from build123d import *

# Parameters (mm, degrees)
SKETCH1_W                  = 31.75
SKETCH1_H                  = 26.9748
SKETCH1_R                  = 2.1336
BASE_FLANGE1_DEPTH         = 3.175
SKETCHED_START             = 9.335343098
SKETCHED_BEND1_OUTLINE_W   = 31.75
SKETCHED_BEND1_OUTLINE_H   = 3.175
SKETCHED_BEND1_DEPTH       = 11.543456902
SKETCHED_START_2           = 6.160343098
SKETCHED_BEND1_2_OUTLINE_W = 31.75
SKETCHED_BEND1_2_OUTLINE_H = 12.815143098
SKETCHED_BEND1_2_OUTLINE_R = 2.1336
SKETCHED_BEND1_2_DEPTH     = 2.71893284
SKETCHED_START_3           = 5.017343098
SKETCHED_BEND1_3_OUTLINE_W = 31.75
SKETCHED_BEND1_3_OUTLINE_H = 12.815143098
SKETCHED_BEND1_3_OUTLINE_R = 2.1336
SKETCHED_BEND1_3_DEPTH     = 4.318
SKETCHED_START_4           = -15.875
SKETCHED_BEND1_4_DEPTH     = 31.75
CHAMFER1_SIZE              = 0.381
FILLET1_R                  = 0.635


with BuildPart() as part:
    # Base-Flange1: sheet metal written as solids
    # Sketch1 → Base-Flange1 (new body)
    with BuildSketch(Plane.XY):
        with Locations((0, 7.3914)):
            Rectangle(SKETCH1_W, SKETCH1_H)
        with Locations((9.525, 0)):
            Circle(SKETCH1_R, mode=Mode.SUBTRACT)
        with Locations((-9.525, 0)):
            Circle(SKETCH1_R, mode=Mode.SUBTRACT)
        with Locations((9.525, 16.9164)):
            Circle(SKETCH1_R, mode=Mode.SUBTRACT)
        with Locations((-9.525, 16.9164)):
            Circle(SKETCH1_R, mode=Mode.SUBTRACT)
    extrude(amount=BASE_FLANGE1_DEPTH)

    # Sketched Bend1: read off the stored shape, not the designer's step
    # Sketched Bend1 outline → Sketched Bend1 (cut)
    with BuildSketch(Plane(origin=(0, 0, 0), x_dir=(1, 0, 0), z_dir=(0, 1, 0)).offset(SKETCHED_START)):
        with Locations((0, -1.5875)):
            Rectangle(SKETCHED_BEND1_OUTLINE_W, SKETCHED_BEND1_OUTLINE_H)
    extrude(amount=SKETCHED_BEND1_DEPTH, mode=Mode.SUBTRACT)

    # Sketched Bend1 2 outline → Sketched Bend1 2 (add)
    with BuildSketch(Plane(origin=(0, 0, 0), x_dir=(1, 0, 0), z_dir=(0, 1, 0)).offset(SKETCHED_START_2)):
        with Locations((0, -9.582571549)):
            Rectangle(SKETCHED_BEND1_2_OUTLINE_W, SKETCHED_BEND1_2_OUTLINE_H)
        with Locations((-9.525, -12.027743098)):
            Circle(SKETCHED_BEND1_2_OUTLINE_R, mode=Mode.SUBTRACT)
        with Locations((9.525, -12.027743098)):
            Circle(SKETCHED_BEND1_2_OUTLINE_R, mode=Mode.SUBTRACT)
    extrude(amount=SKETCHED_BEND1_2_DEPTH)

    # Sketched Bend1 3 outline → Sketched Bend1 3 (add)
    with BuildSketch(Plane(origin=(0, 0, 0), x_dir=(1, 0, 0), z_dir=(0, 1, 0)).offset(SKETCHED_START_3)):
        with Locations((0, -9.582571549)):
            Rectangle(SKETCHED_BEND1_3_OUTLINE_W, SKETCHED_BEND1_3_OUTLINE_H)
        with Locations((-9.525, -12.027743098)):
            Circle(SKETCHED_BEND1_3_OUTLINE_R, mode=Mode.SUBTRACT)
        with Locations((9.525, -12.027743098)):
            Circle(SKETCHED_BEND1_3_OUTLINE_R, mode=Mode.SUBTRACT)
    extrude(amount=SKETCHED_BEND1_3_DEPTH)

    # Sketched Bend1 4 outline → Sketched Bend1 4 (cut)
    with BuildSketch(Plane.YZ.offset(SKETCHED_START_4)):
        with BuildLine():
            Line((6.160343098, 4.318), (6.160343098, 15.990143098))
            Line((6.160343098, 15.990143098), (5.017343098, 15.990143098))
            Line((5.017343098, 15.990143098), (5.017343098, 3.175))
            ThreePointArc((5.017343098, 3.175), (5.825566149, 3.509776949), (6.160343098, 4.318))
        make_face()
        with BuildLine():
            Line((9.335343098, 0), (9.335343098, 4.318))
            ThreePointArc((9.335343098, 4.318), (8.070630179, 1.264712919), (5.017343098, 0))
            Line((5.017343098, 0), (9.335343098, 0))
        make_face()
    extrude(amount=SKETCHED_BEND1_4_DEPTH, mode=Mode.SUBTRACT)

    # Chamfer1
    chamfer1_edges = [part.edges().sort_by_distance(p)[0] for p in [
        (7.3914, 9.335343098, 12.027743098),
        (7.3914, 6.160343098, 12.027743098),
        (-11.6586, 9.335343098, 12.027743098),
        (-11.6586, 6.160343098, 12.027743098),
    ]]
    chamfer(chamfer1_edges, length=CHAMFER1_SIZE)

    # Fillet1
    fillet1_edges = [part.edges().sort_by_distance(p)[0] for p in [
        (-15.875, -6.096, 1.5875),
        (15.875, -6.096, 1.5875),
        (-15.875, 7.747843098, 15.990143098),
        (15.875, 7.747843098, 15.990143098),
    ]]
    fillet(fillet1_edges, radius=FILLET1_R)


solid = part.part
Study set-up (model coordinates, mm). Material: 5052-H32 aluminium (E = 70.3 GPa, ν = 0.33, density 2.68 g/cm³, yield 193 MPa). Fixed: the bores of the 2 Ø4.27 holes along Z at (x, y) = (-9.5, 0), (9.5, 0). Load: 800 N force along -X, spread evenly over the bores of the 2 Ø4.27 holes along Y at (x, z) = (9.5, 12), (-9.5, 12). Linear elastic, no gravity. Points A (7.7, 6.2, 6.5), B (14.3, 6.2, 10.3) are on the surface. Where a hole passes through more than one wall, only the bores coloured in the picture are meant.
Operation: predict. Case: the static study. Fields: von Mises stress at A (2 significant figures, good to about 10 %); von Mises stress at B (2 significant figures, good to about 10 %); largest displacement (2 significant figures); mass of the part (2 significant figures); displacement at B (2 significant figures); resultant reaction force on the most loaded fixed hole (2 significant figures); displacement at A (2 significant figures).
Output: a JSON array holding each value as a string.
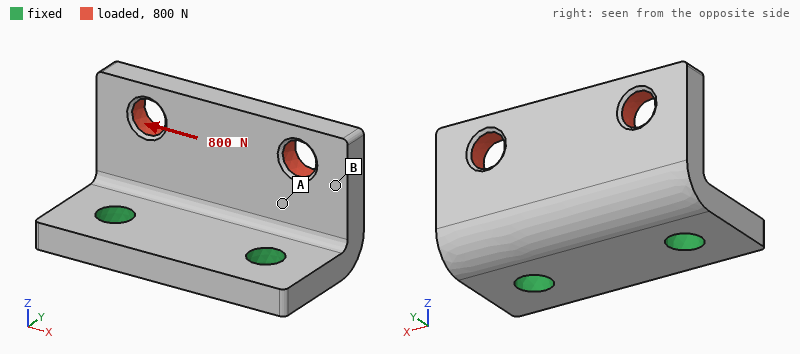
["40 MPa", "20 MPa", "38 µm", "6.8 g", "27 µm", "610 N", "13 µm"]
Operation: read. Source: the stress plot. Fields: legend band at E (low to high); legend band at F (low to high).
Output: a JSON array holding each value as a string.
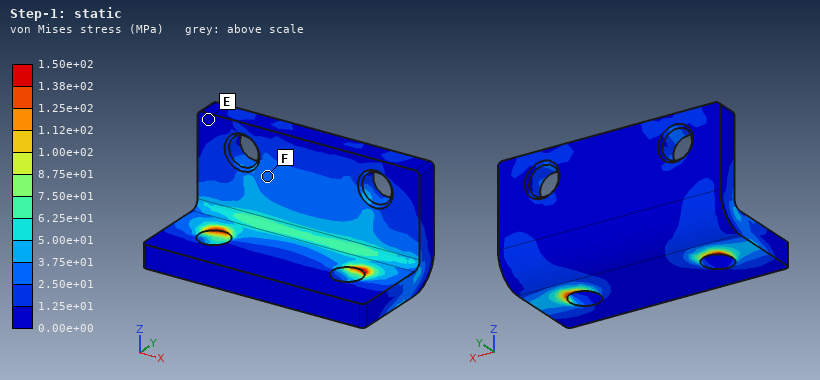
["0.00e+00 to 1.25e+01 MPa", "2.50e+01 to 3.75e+01 MPa"]
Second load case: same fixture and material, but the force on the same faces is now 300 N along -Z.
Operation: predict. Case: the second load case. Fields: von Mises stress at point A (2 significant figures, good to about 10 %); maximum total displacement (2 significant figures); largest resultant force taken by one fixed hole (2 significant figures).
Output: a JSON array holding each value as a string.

["4.6 MPa", "21 µm", "150 N"]
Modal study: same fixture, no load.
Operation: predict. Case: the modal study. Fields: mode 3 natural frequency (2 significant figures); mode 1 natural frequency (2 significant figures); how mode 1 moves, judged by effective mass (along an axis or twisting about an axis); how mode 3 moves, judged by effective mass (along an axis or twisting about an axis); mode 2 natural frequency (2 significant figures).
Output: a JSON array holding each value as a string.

["21 kHz", "7800 Hz", "along Y", "along X", "13 kHz"]
